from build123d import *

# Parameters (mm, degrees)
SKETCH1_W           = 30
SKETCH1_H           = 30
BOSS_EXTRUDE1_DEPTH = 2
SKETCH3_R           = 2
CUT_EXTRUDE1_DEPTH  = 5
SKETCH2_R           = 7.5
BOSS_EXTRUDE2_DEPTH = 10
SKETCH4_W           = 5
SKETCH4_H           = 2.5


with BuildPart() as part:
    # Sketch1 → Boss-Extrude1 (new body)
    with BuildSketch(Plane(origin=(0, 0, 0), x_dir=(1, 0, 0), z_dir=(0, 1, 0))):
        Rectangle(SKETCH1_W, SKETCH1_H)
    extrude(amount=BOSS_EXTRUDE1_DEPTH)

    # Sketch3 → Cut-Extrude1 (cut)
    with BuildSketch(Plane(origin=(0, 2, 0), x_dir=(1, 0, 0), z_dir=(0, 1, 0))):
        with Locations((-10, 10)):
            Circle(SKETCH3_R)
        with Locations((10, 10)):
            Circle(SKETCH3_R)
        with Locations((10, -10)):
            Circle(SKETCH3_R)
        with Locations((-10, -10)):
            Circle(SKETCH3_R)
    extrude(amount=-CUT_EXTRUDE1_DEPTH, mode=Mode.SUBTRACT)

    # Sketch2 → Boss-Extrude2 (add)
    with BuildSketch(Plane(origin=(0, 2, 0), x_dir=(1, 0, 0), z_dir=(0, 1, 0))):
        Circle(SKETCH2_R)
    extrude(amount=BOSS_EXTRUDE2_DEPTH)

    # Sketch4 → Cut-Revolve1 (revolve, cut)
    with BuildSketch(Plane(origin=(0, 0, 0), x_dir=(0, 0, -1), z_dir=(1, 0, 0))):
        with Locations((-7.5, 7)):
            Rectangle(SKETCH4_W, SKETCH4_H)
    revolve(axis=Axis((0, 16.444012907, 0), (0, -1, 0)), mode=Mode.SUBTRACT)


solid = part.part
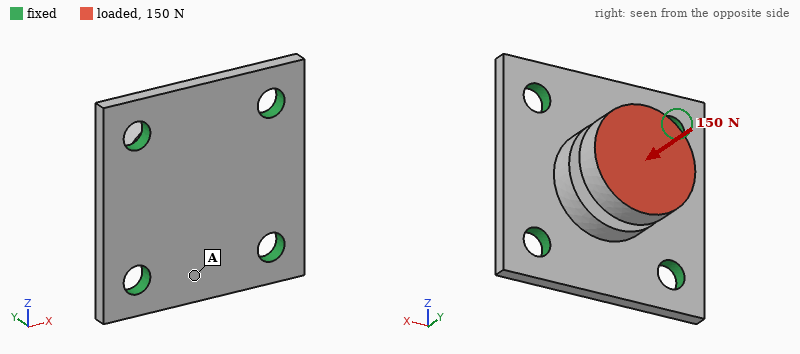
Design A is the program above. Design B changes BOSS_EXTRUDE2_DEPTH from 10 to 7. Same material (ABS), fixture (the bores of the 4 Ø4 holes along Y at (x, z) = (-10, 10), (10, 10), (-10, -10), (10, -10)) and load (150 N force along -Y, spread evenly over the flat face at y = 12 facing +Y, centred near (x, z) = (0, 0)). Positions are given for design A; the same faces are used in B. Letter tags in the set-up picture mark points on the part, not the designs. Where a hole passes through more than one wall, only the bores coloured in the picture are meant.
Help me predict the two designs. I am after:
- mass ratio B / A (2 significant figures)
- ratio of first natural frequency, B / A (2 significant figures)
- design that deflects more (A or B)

0.84
1.2
B
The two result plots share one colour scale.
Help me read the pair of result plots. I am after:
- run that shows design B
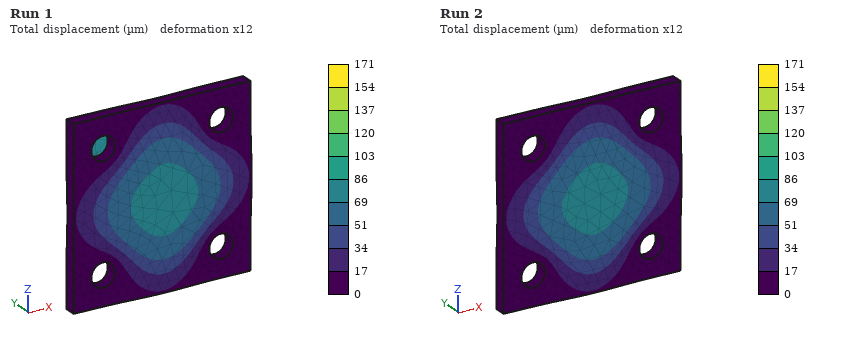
Run 2
